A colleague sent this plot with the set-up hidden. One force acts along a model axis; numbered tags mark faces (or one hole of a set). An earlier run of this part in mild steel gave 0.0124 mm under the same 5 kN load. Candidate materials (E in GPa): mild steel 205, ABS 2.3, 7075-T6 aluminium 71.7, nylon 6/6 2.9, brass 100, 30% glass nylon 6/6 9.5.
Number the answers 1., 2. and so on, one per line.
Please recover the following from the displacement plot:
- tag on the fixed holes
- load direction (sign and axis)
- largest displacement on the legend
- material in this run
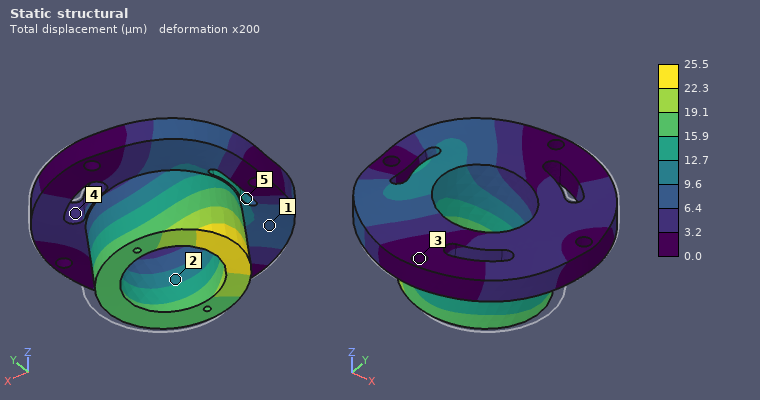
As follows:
1. 3
2. -X
3. 25.5 µm
4. brass
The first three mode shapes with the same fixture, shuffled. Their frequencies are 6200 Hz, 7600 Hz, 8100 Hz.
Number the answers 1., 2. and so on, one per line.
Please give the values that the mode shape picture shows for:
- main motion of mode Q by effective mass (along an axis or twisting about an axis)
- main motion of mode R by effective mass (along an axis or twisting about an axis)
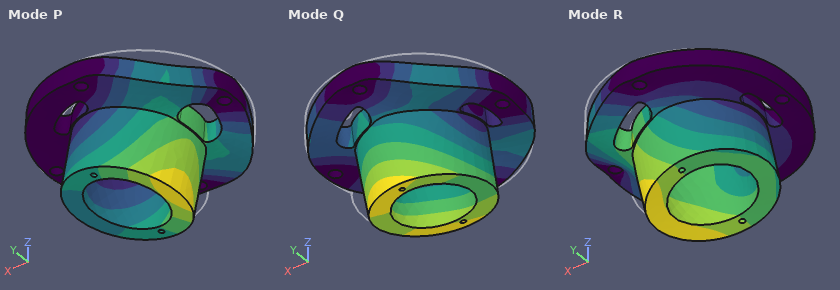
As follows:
1. along Y
2. along Z
